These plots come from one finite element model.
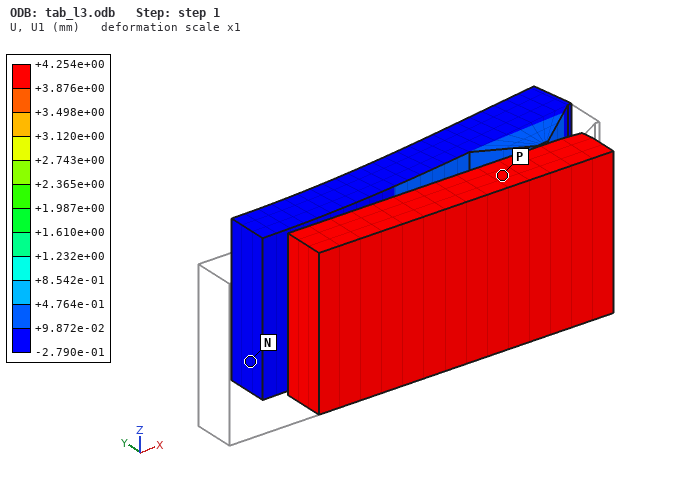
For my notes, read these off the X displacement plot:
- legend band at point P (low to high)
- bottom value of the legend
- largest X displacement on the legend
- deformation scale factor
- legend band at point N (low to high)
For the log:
+3.876e+00 to +4.254e+00 mm
-2.790e-01 mm
+4.254e+00 mm
1
-2.790e-01 to +9.872e-02 mm
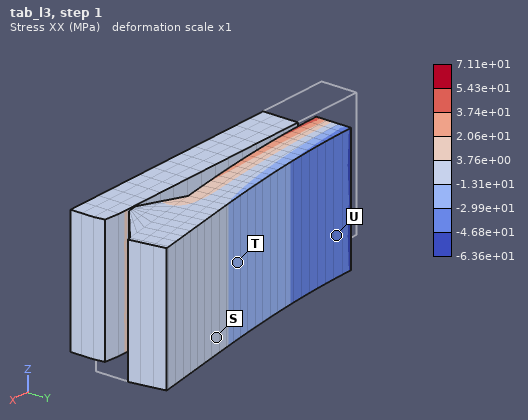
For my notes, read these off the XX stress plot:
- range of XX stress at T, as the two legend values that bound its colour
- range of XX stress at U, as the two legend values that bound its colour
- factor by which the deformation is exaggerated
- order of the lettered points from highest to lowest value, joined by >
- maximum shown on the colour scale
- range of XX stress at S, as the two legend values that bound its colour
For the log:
-2.99e+01 to -1.31e+01 MPa
-4.68e+01 to -2.99e+01 MPa
1
S > T > U
7.11e+01 MPa
-1.31e+01 to 3.76e+00 MPa
